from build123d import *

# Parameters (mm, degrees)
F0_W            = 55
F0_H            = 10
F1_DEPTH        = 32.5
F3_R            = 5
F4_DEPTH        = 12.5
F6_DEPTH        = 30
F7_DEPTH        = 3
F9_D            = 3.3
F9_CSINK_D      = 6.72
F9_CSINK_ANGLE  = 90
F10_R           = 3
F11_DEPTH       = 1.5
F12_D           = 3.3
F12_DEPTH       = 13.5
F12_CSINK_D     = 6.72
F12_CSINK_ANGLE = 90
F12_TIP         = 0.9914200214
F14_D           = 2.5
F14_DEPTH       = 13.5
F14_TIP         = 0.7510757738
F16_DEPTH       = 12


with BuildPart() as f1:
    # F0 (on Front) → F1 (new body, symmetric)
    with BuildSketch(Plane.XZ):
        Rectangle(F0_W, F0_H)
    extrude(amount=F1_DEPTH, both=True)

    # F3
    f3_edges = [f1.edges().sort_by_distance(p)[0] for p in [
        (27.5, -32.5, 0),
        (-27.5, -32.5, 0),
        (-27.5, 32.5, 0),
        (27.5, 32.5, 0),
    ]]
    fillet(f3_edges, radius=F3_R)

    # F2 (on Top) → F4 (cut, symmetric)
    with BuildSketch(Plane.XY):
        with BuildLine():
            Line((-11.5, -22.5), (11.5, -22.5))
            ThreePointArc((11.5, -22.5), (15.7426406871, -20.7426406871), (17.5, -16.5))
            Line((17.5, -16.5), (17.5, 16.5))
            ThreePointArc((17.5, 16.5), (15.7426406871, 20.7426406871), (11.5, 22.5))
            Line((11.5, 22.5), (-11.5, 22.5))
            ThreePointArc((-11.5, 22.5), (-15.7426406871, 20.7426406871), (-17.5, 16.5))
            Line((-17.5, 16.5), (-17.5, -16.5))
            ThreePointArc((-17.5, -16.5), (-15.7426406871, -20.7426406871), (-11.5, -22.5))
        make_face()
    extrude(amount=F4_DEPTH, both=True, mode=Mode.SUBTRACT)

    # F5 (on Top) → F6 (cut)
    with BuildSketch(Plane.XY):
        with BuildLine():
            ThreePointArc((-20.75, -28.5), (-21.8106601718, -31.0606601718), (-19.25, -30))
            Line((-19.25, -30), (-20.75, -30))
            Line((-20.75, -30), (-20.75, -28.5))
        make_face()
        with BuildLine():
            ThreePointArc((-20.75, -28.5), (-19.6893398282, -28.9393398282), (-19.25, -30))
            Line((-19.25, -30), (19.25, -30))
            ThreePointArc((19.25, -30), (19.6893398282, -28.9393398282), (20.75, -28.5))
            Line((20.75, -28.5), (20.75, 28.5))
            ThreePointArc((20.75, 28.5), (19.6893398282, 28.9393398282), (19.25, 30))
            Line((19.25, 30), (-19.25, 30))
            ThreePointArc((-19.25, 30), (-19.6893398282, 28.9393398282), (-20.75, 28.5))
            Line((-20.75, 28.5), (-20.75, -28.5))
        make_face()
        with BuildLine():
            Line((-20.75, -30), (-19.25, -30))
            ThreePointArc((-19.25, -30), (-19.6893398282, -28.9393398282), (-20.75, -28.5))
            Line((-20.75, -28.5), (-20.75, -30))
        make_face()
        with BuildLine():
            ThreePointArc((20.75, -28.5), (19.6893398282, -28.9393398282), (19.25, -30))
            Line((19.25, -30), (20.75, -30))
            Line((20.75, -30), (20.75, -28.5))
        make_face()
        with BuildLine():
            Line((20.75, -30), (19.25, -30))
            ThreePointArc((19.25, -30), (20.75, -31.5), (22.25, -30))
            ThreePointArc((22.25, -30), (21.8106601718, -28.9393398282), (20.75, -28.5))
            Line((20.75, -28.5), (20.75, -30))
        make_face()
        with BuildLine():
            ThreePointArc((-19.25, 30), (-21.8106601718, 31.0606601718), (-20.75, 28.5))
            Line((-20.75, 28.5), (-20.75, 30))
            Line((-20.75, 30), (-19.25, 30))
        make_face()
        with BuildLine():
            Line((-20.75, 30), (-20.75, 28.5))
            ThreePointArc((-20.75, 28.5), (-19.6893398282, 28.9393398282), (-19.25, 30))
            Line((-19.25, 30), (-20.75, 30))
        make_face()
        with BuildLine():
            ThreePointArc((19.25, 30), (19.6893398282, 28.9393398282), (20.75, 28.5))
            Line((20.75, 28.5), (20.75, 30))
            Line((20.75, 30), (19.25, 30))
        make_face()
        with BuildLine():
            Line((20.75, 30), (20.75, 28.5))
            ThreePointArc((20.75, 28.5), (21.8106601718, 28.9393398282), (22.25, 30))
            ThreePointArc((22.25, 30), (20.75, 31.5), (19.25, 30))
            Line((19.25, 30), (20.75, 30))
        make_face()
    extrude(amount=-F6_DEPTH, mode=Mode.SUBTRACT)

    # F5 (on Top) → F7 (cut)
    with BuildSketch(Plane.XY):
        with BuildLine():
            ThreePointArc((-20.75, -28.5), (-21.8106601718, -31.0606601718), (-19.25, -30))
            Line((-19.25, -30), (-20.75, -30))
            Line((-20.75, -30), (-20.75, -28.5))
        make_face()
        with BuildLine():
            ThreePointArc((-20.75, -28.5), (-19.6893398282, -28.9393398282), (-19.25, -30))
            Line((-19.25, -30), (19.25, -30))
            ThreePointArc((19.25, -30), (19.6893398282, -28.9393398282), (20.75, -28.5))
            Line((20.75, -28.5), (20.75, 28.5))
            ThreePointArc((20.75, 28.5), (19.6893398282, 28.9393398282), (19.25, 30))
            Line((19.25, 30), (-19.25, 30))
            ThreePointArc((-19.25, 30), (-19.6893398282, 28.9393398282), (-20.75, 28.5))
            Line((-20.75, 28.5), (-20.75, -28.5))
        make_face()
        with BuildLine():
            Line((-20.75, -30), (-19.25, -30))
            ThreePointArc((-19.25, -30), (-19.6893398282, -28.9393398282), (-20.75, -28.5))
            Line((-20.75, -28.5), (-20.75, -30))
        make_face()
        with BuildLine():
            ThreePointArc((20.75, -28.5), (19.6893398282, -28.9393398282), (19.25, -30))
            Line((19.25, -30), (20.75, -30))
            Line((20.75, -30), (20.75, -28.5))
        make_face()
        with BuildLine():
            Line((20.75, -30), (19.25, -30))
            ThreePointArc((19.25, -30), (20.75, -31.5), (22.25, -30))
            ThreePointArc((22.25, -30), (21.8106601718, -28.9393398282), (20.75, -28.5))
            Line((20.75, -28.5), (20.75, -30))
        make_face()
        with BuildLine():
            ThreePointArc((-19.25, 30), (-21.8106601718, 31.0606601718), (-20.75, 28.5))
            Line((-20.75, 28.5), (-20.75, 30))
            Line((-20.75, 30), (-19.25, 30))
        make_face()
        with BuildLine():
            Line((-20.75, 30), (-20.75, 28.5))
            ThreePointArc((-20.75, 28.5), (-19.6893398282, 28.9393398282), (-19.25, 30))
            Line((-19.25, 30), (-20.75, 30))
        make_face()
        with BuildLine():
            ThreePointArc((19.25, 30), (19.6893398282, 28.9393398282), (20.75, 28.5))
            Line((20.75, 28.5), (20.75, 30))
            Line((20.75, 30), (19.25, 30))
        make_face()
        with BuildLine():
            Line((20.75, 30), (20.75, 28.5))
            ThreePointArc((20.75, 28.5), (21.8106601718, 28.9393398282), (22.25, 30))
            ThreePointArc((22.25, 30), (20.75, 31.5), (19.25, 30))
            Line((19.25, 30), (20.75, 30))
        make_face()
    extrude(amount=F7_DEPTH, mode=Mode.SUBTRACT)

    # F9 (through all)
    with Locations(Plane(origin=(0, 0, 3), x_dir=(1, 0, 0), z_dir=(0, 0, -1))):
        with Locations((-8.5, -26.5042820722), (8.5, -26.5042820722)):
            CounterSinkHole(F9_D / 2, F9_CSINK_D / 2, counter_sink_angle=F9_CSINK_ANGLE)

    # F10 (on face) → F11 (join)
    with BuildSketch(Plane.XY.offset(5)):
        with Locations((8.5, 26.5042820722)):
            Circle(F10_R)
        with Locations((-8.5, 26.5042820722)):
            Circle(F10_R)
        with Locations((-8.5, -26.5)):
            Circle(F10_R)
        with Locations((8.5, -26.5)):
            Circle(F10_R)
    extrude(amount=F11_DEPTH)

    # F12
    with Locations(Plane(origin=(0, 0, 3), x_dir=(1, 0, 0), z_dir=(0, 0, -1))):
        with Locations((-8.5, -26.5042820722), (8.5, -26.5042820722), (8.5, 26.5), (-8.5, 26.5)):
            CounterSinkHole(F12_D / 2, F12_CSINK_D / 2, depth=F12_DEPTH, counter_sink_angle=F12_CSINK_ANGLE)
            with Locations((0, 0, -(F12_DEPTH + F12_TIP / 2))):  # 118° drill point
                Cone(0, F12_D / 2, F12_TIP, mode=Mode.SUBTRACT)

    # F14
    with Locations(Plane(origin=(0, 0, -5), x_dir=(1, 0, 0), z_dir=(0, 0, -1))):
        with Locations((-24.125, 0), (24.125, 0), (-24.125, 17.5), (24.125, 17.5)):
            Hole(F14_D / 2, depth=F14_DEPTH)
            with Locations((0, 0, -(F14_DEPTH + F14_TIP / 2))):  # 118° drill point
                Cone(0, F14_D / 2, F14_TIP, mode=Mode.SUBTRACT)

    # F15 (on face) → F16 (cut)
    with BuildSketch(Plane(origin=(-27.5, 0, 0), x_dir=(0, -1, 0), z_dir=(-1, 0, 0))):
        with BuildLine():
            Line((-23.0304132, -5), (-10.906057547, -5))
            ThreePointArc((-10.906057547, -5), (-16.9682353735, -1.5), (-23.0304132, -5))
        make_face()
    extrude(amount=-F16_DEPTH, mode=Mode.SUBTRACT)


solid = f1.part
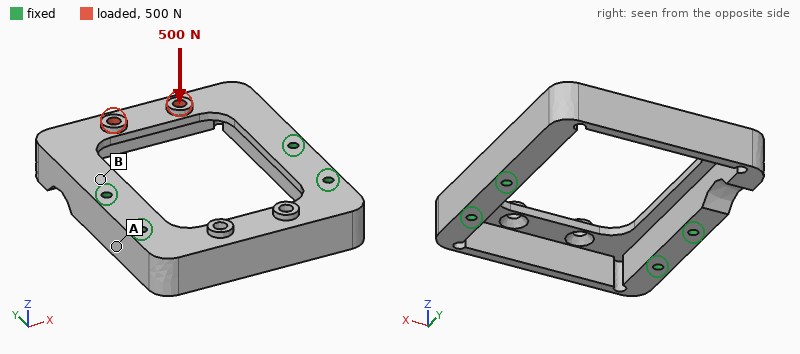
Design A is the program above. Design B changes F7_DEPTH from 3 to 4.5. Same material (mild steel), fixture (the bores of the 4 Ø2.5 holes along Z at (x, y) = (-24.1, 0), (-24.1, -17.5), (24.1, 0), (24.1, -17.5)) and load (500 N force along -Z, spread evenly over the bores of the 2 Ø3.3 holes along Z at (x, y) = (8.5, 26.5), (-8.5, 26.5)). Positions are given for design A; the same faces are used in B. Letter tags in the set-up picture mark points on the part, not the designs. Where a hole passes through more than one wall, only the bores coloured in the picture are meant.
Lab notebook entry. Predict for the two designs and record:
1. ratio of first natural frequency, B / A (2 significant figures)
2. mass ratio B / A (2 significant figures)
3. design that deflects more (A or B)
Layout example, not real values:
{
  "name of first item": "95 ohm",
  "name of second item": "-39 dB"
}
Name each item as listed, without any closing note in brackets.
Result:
{
  "ratio of first natural frequency, B / A": "1.0",
  "mass ratio B / A": "0.89",
  "design that deflects more": "B"
}
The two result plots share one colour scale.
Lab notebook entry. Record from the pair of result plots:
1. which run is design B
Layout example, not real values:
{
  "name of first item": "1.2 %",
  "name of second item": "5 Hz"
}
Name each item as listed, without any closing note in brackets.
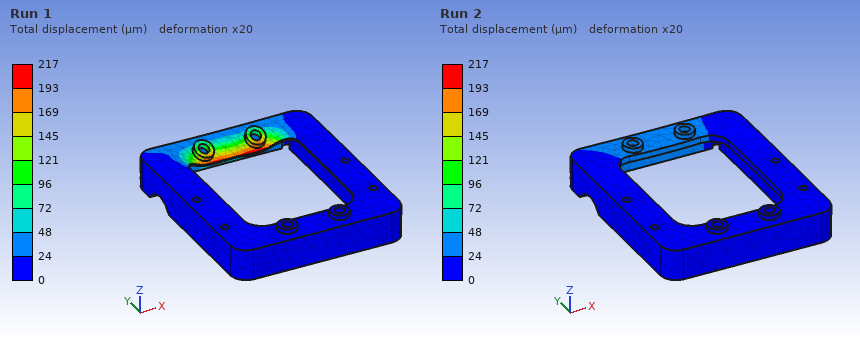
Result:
{
  "which run is design B": "Run 1"
}
